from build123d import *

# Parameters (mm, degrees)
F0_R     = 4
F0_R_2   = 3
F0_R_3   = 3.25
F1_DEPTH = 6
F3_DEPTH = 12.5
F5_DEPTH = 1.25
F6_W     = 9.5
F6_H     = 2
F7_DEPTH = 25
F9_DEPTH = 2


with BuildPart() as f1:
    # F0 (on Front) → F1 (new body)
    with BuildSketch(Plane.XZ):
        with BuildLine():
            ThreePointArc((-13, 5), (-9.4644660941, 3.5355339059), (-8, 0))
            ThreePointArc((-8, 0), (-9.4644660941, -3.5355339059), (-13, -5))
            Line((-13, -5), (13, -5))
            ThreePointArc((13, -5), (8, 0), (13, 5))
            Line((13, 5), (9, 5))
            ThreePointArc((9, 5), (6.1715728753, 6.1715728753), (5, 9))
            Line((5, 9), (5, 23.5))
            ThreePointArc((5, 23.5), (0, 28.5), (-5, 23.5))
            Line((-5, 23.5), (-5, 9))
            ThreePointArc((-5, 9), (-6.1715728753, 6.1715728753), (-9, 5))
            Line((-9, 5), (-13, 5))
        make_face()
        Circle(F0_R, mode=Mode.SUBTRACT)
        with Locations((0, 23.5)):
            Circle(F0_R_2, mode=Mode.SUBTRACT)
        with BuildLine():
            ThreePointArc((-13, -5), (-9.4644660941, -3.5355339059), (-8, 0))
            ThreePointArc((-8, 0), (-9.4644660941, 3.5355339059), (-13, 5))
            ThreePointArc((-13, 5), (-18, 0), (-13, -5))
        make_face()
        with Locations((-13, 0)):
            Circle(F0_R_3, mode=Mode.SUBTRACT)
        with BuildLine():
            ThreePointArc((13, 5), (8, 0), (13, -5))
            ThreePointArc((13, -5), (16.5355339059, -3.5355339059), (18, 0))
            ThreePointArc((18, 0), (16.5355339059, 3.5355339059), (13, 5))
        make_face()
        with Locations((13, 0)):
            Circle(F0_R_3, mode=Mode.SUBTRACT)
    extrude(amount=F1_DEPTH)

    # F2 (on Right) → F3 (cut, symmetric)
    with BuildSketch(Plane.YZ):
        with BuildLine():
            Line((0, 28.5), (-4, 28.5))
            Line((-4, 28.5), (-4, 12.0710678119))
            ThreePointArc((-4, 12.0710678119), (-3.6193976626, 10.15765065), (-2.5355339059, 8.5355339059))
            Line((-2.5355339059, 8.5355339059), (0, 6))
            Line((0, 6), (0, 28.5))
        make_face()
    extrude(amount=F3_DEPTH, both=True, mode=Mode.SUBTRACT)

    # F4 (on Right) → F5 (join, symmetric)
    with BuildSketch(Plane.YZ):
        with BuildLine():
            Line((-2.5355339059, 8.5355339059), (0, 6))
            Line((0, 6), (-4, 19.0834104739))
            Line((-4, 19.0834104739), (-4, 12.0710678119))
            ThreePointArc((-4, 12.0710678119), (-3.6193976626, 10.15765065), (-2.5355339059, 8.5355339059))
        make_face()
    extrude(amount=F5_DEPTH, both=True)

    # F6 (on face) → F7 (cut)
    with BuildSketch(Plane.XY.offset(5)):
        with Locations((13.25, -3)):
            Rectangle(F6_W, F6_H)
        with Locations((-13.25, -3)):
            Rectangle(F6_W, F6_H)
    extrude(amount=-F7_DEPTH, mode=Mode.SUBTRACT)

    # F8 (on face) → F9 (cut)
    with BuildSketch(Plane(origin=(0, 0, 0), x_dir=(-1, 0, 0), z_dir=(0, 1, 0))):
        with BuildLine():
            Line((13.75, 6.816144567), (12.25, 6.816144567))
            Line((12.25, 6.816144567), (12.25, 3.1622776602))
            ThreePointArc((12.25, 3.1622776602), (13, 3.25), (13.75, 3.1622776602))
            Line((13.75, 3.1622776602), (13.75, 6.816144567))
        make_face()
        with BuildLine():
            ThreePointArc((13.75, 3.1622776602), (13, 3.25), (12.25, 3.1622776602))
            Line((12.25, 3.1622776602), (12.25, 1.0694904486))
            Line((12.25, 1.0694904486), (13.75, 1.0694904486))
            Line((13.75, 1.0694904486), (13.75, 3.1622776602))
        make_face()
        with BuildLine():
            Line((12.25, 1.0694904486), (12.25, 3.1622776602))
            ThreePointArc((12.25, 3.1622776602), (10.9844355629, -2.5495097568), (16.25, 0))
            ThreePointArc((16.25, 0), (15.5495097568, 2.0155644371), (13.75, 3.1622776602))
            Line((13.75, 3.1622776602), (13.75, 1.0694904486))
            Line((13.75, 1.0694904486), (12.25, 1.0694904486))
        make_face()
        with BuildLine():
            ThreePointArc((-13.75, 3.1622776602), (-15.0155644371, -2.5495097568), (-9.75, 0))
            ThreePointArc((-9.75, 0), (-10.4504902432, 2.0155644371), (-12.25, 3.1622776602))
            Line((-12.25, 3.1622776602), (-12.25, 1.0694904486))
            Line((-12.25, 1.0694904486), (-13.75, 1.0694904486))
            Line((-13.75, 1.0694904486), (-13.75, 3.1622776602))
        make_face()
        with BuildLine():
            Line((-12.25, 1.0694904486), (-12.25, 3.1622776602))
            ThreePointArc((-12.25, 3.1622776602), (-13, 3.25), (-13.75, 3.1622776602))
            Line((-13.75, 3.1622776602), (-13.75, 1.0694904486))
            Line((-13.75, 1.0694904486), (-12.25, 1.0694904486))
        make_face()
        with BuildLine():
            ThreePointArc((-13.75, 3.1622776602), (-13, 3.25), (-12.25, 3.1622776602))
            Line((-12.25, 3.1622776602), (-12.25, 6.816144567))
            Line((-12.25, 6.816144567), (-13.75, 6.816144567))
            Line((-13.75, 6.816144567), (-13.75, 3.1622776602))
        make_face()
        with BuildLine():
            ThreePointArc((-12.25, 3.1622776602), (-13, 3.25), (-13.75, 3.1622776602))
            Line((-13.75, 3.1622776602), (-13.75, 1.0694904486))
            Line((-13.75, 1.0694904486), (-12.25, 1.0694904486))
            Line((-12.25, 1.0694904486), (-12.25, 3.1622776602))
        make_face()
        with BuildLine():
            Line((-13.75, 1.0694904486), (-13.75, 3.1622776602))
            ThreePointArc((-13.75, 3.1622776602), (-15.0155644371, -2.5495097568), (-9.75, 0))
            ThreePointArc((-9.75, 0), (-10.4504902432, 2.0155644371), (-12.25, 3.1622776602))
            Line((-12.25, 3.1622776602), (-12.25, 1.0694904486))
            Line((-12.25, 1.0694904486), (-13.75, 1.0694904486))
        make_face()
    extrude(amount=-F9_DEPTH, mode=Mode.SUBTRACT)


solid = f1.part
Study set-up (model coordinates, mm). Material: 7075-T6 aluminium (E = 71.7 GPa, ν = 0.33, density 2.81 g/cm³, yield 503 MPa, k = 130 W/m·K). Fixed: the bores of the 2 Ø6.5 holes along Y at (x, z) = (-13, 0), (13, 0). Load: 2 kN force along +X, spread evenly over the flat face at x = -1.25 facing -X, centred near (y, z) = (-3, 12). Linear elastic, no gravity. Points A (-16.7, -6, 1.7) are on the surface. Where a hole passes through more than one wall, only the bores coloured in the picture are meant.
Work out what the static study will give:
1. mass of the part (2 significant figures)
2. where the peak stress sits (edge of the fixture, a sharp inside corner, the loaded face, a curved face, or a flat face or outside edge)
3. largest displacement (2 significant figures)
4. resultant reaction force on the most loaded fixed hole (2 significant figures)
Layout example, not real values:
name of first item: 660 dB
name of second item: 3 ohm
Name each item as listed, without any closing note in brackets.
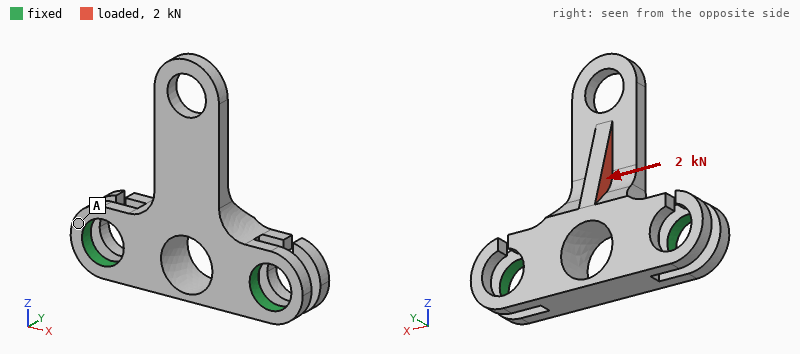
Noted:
mass of the part: 4.8 g
where the peak stress sits: a curved face
largest displacement: 0.13 mm
resultant reaction force on the most loaded fixed hole: 1.6 kN
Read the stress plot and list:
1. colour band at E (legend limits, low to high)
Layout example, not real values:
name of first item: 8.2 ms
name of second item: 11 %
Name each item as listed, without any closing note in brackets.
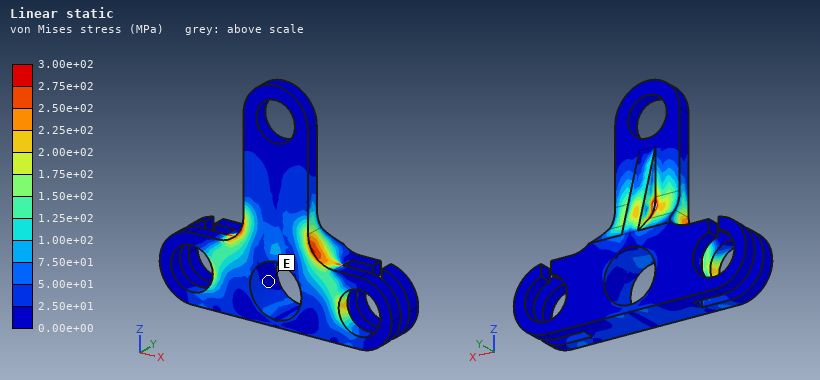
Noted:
colour band at E: 0.00e+00 to 2.50e+01 MPa
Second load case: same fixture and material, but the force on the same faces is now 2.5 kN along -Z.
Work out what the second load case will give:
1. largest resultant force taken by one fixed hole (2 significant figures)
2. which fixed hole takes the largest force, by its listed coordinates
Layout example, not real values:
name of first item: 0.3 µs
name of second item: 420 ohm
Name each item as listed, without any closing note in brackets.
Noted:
largest resultant force taken by one fixed hole: 1.5 kN
which fixed hole takes the largest force, by its listed coordinates: (-13, 0)
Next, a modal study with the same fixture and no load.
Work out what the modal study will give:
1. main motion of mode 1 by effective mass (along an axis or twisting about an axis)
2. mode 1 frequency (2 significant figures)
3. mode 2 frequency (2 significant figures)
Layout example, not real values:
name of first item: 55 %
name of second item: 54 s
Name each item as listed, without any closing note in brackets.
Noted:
main motion of mode 1 by effective mass: along Y
mode 1 frequency: 5700 Hz
mode 2 frequency: 7200 Hz
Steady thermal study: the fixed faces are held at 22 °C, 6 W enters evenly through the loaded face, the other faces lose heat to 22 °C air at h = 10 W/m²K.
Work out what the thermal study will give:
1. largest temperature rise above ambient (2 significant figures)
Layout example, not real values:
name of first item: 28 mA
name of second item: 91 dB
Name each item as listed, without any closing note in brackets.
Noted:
largest temperature rise above ambient: 19 K
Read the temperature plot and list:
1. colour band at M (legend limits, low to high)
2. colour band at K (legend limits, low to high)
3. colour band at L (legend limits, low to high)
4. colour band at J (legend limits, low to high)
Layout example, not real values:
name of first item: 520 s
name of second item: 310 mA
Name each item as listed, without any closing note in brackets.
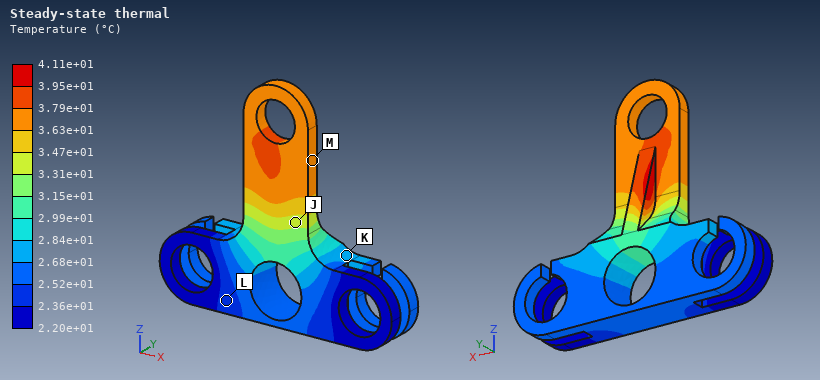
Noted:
colour band at M: 3.63e+01 to 3.79e+01 °C
colour band at K: 2.68e+01 to 2.84e+01 °C
colour band at L: 2.36e+01 to 2.52e+01 °C
colour band at J: 3.31e+01 to 3.47e+01 °C
